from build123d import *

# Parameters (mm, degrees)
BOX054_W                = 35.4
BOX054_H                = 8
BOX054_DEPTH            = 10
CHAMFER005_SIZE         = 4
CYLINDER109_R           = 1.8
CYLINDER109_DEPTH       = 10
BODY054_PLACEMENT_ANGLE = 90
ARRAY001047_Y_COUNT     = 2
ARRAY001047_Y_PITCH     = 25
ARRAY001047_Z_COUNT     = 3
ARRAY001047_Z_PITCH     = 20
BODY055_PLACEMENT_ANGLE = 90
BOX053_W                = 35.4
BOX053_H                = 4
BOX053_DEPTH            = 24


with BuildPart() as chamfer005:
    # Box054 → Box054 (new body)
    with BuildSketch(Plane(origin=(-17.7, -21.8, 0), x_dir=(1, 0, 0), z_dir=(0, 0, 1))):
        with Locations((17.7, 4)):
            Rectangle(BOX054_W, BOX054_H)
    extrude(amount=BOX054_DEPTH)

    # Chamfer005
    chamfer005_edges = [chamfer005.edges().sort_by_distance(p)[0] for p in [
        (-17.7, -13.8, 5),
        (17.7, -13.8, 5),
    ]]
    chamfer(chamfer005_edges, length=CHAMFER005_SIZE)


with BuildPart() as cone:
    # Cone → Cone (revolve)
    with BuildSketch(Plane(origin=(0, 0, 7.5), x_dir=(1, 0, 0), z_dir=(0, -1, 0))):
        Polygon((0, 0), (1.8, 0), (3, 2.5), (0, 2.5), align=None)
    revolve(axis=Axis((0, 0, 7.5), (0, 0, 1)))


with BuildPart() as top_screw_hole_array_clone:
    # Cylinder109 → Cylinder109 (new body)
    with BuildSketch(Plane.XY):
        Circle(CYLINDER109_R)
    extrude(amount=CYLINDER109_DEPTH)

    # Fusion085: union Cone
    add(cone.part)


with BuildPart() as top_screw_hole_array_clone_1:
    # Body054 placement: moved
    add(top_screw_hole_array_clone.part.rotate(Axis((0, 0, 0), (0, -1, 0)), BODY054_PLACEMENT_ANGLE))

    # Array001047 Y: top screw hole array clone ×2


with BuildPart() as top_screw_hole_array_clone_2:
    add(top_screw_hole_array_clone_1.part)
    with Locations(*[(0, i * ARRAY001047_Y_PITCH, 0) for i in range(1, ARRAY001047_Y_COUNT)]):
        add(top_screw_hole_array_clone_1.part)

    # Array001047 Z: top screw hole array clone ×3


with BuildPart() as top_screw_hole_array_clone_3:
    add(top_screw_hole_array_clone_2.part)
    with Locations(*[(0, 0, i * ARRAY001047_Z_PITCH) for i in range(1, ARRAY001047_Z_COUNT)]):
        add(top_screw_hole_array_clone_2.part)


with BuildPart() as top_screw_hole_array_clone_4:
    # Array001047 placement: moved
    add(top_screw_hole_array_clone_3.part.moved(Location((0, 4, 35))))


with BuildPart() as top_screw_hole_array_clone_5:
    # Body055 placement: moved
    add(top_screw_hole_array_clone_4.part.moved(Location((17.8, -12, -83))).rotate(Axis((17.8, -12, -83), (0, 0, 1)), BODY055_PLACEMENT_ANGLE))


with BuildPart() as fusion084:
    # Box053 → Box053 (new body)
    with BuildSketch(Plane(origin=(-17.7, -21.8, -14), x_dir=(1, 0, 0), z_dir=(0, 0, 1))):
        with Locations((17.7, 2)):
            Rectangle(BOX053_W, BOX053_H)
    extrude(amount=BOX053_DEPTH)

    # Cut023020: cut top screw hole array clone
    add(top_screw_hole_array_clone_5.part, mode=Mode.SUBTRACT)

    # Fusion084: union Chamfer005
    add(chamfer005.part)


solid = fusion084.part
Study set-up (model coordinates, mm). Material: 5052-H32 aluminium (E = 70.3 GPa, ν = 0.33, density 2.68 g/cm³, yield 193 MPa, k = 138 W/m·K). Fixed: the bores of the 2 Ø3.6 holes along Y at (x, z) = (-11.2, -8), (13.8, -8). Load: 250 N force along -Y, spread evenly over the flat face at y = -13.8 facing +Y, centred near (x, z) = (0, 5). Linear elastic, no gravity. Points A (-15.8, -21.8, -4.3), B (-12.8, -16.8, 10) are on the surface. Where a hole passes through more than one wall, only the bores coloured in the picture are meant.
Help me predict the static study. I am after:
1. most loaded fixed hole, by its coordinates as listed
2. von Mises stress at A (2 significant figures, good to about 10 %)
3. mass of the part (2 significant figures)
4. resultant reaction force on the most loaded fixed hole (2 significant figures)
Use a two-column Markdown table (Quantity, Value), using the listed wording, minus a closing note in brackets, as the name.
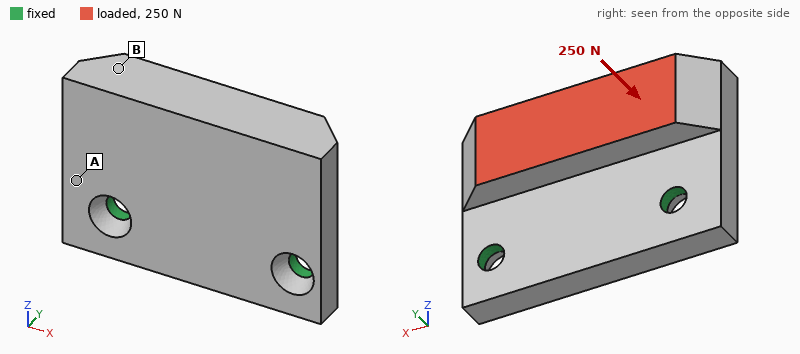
| Quantity | Value |
|---|---|
| most loaded fixed hole, by its coordinates as listed | (-11.2, -8) |
| von Mises stress at A | 33 MPa |
| mass of the part | 12 g |
| resultant reaction force on the most loaded fixed hole | 140 N |
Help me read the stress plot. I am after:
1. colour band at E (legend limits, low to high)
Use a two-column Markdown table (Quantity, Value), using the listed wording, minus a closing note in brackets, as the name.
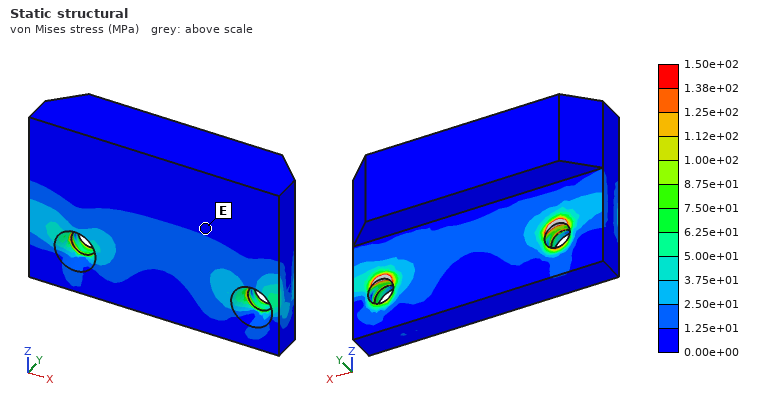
| Quantity | Value |
|---|---|
| colour band at E | 0.00e+00 to 1.25e+01 MPa |
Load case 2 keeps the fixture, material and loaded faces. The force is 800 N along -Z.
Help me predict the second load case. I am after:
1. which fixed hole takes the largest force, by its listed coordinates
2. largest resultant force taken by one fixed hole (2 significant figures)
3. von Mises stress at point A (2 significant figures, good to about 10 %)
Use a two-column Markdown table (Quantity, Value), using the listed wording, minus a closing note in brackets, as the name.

| Quantity | Value |
|---|---|
| which fixed hole takes the largest force, by its listed coordinates | (-11.2, -8) |
| largest resultant force taken by one fixed hole | 450 N |
| von Mises stress at point A | 56 MPa |
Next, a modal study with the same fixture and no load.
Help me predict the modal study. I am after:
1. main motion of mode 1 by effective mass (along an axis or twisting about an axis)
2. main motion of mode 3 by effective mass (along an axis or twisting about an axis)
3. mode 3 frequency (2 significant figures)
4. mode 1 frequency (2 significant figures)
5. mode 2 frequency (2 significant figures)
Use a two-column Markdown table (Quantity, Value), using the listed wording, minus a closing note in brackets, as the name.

| Quantity | Value |
|---|---|
| main motion of mode 1 by effective mass | along Y |
| main motion of mode 3 by effective mass | along X |
| mode 3 frequency | 23 kHz |
| mode 1 frequency | 4700 Hz |
| mode 2 frequency | 13 kHz |
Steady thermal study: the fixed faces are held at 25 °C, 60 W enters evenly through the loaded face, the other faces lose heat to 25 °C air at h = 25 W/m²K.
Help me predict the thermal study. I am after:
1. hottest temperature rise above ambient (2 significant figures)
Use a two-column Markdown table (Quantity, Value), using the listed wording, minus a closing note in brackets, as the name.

| Quantity | Value |
|---|---|
| hottest temperature rise above ambient | 54 K |
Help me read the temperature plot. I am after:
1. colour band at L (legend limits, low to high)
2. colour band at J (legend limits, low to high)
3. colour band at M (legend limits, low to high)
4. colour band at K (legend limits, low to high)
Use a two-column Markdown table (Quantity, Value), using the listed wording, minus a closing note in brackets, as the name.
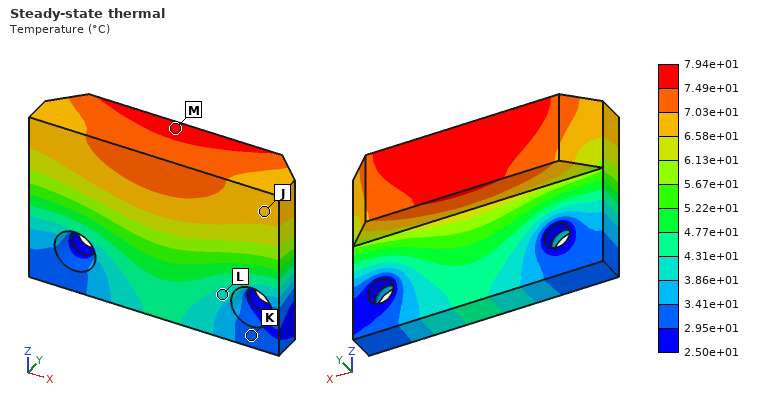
| Quantity | Value |
|---|---|
| colour band at L | 3.86e+01 to 4.31e+01 °C |
| colour band at J | 6.58e+01 to 7.03e+01 °C |
| colour band at M | 7.49e+01 to 7.94e+01 °C |
| colour band at K | 2.95e+01 to 3.41e+01 °C |
